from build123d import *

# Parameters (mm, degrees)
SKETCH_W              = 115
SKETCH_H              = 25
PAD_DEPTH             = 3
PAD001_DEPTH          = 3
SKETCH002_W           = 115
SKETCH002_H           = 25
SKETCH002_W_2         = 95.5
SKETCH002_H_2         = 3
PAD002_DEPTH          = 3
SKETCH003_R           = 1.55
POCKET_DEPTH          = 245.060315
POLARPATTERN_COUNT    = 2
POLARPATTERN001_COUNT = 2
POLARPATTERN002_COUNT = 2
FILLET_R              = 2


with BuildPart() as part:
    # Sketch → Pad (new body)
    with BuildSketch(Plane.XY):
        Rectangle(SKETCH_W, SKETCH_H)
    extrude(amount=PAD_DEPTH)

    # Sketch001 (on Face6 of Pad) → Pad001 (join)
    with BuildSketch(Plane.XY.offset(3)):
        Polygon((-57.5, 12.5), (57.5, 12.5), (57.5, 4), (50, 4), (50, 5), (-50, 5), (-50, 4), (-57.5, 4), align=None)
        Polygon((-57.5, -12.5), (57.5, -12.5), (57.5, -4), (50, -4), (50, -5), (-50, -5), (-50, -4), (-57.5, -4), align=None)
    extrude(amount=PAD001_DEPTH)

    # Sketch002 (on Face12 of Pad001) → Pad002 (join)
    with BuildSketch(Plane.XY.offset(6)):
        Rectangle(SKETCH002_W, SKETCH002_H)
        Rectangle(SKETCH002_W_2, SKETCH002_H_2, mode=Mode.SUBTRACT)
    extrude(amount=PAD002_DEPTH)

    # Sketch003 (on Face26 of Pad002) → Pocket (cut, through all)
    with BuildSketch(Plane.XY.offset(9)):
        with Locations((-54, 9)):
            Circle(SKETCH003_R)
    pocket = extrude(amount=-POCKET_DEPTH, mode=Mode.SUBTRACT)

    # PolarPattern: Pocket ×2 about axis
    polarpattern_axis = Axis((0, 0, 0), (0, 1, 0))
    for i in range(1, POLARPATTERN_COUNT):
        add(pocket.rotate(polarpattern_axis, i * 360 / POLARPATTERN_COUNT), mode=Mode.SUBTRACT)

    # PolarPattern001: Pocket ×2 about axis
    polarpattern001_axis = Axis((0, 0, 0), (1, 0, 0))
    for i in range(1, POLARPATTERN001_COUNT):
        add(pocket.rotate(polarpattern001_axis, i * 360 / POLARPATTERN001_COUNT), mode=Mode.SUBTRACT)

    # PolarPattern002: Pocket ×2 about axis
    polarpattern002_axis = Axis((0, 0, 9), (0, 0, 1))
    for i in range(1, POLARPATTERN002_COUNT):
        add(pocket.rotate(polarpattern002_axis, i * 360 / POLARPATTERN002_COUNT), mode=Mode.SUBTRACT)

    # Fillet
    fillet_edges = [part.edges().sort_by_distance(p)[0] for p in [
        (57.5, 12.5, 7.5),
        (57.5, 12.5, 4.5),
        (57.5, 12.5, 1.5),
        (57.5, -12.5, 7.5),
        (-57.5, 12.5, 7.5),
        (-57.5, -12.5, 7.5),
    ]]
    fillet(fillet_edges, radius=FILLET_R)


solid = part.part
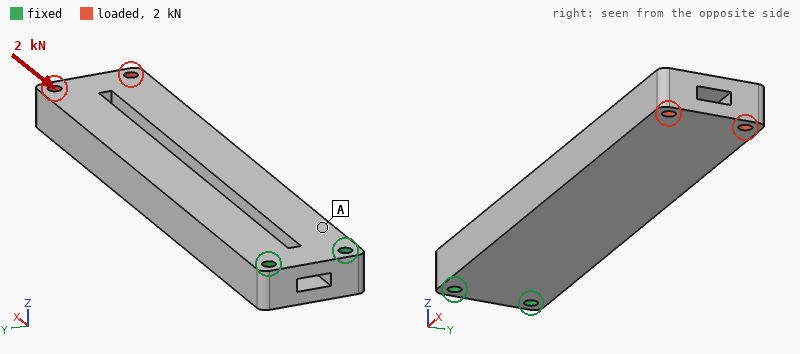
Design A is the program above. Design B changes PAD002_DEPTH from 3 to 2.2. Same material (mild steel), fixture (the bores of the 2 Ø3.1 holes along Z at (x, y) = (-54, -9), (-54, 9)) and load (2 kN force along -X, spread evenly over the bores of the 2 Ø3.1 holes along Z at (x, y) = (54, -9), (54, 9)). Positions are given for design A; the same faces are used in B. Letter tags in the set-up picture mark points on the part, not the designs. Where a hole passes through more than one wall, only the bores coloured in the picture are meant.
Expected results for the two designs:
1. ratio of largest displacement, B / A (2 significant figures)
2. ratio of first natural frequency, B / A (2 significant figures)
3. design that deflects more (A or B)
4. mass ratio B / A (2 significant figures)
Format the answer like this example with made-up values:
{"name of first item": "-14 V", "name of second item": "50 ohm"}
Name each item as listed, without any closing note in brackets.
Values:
{"ratio of largest displacement, B / A": "1.4", "ratio of first natural frequency, B / A": "0.91", "design that deflects more": "B", "mass ratio B / A": "0.90"}
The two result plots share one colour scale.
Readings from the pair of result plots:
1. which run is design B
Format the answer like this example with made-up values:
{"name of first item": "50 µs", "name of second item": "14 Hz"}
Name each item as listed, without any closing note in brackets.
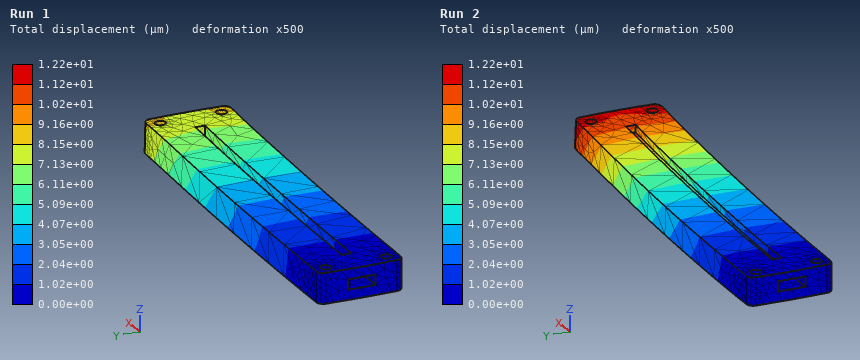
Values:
{"which run is design B": "Run 2"}
